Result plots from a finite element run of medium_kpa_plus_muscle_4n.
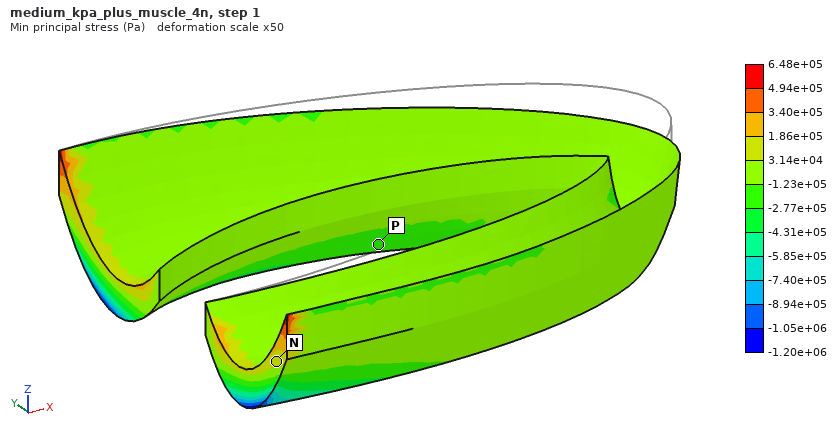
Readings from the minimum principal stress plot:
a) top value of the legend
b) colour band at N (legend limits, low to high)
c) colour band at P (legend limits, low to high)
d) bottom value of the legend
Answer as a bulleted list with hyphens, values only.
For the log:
- 6.48e+05 Pa
- 3.14e+04 to 1.86e+05 Pa
- -2.77e+05 to -1.23e+05 Pa
- -1.20e+06 Pa
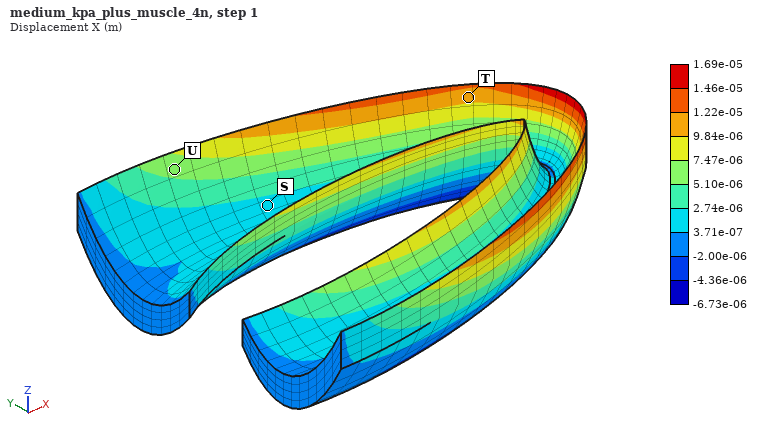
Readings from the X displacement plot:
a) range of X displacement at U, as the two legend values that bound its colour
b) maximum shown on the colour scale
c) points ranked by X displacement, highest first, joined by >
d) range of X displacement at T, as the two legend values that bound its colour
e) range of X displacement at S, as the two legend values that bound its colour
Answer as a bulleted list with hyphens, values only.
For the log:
- 5.10e-06 to 7.47e-06 m
- 1.69e-05 m
- T > U > S
- 9.84e-06 to 1.22e-05 m
- 3.71e-07 to 2.74e-06 m
